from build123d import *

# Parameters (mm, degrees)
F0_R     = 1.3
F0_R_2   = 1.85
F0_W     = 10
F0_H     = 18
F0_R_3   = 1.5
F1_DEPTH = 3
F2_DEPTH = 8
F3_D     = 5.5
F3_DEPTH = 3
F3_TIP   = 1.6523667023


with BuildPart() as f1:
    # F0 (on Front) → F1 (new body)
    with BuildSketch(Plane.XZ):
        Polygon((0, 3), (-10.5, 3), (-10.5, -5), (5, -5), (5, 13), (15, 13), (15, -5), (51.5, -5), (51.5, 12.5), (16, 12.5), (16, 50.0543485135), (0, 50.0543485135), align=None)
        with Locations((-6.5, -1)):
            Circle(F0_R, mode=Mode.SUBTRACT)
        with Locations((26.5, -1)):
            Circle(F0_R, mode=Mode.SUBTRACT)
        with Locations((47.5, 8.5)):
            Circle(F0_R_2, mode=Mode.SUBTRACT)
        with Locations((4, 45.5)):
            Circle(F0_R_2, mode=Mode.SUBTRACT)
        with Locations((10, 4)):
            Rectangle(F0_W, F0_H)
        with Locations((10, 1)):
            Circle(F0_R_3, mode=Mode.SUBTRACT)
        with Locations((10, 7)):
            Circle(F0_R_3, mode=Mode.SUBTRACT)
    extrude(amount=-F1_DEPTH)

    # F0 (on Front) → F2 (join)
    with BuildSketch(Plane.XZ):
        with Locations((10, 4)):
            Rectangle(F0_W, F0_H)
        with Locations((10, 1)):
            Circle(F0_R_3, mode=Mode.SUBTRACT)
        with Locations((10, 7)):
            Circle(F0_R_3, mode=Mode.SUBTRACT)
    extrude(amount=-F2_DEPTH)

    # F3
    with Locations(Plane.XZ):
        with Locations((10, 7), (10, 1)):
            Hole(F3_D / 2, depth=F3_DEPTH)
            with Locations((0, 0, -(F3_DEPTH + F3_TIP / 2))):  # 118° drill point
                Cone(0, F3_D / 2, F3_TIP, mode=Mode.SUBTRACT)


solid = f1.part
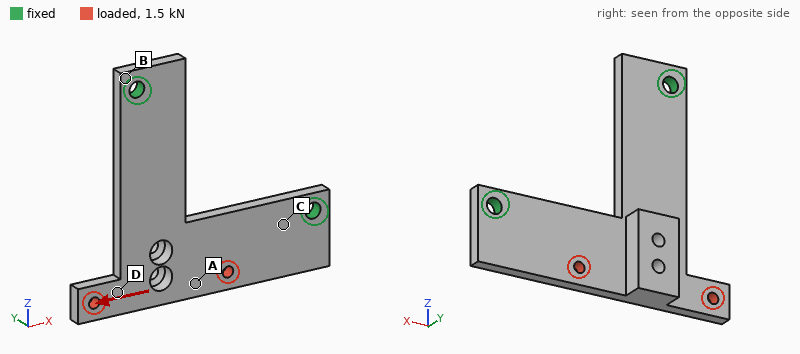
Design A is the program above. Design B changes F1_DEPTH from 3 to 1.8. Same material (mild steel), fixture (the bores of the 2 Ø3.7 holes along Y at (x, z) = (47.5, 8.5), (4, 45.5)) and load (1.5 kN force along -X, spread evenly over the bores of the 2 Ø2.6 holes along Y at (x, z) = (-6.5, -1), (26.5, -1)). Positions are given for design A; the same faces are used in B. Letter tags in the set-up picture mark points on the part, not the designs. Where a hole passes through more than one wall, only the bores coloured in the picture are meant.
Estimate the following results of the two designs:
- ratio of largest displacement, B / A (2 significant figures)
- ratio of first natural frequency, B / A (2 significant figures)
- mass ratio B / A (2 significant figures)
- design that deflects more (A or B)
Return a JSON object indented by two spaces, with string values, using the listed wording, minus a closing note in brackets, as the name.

{
  "ratio of largest displacement, B / A": "1.6",
  "ratio of first natural frequency, B / A": "0.55",
  "mass ratio B / A": "0.69",
  "design that deflects more": "B"
}
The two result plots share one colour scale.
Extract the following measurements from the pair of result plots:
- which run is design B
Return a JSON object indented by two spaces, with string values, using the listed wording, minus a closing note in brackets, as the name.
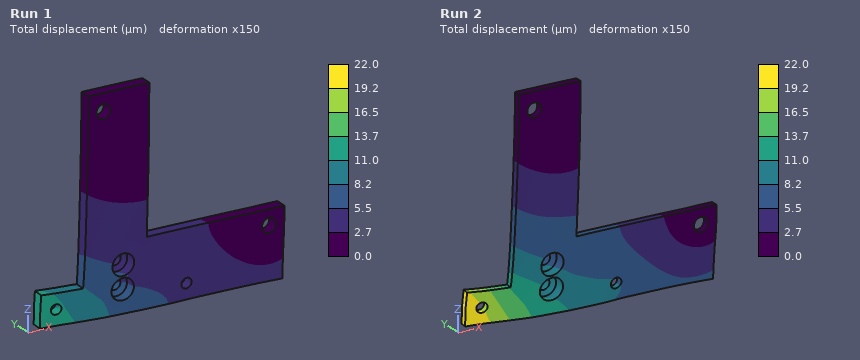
{
  "which run is design B": "Run 2"
}
